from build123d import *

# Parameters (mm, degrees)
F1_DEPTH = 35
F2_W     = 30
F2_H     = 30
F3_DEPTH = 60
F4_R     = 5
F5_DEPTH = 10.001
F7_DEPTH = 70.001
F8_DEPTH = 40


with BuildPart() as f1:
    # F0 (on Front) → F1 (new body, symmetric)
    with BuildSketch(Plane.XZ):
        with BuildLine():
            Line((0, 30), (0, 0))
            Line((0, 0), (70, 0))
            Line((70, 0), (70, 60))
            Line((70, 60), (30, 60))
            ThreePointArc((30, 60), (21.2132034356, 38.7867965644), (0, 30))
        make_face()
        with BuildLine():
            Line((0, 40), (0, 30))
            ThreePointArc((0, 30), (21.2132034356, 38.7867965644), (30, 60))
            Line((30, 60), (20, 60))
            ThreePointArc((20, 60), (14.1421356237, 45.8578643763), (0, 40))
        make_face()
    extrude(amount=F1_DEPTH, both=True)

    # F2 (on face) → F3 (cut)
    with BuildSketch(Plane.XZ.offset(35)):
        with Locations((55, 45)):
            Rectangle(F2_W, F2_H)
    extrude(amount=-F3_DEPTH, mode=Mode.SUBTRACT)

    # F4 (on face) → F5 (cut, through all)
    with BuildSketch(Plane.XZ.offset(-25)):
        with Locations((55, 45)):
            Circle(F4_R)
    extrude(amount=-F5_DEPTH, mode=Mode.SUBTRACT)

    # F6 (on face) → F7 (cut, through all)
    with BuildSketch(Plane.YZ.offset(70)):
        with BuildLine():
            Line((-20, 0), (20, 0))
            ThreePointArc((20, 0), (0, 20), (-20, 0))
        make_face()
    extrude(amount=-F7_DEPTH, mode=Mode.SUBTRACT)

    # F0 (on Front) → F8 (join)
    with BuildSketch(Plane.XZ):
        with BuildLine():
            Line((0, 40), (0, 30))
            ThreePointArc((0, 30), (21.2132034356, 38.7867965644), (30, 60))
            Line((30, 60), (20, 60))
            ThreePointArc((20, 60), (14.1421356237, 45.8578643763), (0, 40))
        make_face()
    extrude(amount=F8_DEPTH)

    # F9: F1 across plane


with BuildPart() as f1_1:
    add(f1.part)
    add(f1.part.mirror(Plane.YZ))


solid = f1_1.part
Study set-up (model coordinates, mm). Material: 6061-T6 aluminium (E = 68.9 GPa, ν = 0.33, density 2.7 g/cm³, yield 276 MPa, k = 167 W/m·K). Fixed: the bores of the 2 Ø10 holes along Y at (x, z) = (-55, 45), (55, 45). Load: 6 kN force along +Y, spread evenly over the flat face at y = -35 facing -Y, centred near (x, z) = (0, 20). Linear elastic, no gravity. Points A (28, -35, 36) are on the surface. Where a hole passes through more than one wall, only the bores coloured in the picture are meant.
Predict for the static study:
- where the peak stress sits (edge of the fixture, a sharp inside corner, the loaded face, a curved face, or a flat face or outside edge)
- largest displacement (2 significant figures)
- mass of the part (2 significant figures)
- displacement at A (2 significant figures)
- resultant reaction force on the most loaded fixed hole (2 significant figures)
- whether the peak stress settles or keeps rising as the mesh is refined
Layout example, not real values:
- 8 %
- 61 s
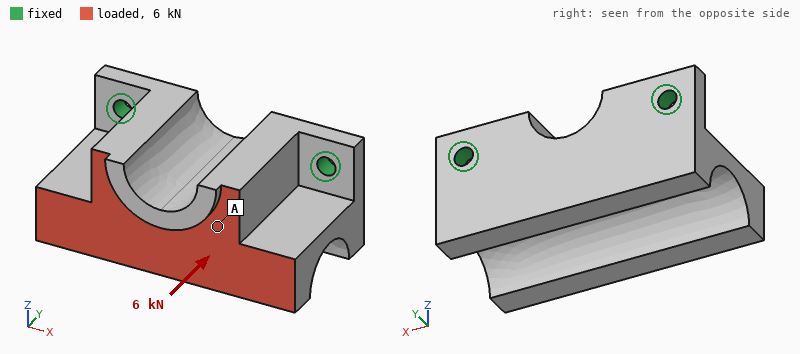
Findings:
- edge of the fixture
- 0.17 mm
- 950 g
- 0.14 mm
- 3.0 kN
- keeps rising
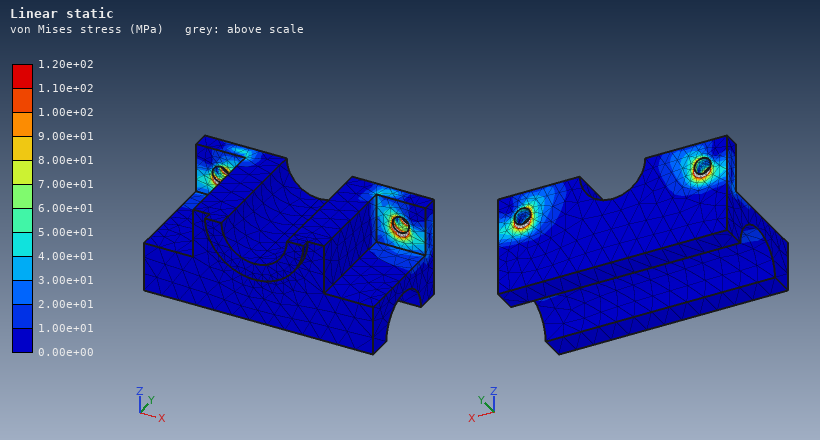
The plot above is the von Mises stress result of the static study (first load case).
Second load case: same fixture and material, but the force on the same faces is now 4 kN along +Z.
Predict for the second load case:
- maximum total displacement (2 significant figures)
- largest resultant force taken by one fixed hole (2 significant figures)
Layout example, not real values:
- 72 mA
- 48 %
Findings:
- 0.35 mm
- 2.5 kN
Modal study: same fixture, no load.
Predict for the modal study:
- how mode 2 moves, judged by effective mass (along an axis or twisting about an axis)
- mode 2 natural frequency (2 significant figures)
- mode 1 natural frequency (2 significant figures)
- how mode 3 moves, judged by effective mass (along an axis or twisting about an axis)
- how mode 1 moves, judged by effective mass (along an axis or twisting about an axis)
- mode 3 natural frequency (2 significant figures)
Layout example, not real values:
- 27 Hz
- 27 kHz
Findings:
- along X
- 3400 Hz
- 940 Hz
- along X
- along Z
- 4000 Hz
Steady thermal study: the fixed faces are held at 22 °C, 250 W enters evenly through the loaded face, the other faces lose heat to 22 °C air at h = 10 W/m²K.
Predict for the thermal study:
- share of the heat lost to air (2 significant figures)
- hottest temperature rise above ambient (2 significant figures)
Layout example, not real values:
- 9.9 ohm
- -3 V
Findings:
- 6.1 %
- 57 K
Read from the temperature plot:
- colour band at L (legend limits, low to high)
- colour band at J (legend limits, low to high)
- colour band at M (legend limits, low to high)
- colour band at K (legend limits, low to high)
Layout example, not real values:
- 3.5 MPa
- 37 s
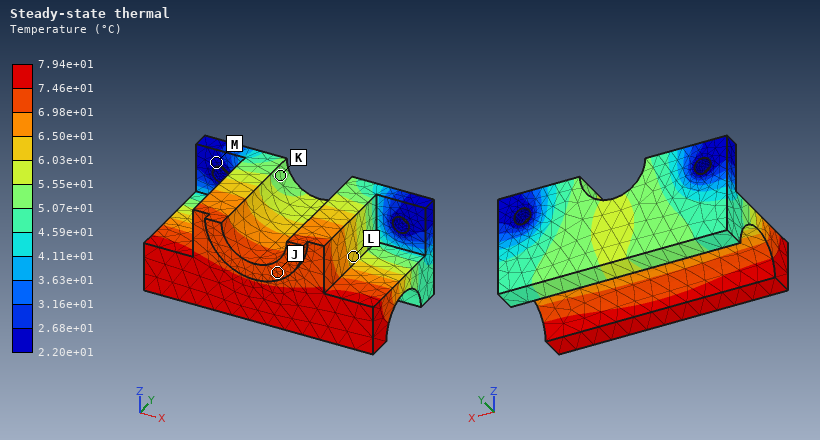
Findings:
- 6.03e+01 to 6.50e+01 °C
- 6.98e+01 to 7.46e+01 °C
- 2.20e+01 to 2.68e+01 °C
- 5.07e+01 to 5.55e+01 °C
